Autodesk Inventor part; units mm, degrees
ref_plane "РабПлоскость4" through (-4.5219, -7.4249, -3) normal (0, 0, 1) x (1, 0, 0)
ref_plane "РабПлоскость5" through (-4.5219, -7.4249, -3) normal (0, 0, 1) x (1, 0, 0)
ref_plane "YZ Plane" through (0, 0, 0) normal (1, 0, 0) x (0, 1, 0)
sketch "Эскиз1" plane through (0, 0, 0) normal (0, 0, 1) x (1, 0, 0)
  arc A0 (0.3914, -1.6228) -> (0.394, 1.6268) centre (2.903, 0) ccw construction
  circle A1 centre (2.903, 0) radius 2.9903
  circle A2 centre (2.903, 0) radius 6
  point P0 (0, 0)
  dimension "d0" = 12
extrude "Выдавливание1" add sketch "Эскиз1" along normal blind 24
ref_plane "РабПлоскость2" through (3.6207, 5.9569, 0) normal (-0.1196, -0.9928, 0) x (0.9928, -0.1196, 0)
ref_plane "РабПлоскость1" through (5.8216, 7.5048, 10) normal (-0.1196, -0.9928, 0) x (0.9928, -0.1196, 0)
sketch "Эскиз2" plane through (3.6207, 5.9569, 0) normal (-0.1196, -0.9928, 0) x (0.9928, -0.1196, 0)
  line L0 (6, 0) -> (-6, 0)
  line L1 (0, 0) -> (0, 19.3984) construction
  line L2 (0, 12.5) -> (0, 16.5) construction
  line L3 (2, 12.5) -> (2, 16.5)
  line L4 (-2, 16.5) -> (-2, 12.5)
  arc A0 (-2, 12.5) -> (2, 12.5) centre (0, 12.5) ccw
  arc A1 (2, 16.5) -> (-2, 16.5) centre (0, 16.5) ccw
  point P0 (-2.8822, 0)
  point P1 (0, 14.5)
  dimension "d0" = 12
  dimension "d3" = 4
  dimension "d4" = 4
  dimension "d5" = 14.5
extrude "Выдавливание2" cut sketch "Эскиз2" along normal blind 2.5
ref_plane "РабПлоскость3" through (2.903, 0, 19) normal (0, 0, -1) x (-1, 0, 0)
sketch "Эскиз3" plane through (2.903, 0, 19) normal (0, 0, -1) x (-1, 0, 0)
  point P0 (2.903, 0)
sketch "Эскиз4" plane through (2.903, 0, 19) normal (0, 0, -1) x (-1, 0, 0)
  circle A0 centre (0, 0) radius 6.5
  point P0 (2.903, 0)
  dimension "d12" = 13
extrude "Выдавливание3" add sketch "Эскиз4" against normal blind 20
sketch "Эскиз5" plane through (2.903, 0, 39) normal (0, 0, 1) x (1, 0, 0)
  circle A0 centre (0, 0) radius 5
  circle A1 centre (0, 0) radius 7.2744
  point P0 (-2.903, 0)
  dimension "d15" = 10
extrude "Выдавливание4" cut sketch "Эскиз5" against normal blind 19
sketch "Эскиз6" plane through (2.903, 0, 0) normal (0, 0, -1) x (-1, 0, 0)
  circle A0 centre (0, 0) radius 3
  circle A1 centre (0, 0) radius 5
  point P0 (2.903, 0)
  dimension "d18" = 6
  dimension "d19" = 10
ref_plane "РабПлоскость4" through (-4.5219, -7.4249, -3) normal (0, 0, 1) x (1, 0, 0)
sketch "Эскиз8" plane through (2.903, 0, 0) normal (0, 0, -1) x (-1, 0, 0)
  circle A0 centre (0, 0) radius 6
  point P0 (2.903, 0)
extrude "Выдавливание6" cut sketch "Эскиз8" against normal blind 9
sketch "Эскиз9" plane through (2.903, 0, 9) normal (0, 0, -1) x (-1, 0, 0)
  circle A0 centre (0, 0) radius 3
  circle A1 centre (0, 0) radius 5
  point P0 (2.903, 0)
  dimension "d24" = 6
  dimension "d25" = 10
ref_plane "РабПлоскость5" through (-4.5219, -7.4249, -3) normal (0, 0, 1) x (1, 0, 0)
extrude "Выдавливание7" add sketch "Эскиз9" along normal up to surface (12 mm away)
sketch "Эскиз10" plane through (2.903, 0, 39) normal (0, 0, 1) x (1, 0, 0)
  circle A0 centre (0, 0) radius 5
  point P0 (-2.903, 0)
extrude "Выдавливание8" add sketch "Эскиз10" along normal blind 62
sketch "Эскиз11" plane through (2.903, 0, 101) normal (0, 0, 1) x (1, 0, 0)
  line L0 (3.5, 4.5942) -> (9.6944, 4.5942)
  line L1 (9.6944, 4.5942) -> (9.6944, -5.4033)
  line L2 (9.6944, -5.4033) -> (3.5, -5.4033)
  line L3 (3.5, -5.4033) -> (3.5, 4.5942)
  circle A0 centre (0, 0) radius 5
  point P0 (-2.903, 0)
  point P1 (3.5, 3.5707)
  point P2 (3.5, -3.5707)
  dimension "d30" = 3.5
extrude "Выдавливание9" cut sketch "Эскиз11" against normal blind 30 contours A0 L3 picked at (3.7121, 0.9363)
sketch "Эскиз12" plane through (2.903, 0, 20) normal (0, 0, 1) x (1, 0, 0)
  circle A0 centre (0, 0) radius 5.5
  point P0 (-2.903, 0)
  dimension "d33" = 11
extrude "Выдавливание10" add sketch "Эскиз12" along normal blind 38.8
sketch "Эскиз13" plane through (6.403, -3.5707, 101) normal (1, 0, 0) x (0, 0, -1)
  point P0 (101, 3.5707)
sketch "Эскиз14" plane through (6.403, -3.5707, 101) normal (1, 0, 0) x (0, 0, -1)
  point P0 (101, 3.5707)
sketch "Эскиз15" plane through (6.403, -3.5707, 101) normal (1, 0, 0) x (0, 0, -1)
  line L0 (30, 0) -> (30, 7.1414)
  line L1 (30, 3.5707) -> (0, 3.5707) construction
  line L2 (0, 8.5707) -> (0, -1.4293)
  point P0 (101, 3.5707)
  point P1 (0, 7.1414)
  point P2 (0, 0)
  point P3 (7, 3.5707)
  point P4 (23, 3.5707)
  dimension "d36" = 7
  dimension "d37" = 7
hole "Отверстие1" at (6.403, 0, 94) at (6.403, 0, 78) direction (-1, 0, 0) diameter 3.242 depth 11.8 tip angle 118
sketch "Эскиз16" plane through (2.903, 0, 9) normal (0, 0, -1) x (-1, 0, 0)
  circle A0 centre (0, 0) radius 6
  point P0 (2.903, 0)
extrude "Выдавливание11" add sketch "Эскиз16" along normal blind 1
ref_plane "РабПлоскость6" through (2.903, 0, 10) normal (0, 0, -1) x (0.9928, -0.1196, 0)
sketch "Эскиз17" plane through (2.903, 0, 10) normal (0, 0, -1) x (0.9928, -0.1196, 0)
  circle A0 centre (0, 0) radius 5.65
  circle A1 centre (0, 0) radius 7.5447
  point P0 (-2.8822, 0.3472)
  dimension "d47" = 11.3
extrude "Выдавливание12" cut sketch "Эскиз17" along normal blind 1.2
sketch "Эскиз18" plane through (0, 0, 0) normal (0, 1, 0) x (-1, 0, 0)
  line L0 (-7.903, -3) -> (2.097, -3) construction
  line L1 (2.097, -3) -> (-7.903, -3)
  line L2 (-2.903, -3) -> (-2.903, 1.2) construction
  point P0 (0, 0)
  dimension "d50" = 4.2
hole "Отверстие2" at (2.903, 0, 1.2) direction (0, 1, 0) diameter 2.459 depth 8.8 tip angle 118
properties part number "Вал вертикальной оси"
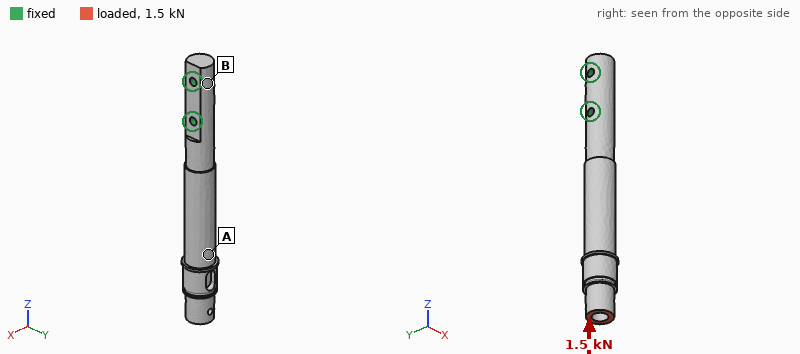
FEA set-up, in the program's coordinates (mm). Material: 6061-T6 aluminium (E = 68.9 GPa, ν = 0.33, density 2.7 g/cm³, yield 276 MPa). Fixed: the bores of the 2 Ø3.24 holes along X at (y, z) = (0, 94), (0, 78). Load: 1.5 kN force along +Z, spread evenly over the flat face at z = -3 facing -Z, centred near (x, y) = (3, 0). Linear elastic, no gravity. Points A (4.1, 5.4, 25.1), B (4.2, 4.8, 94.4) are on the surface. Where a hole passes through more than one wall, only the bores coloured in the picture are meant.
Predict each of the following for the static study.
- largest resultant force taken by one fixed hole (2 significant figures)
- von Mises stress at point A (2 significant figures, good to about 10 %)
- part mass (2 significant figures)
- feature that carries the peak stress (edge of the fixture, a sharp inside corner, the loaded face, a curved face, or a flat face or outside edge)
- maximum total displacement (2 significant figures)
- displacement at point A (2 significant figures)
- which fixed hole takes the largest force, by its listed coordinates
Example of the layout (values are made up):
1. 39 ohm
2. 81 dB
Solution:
1. 1.4 kN
2. 15 MPa
3. 22 g
4. a curved face
5. 32 µm
6. 18 µm
7. (0, 78)
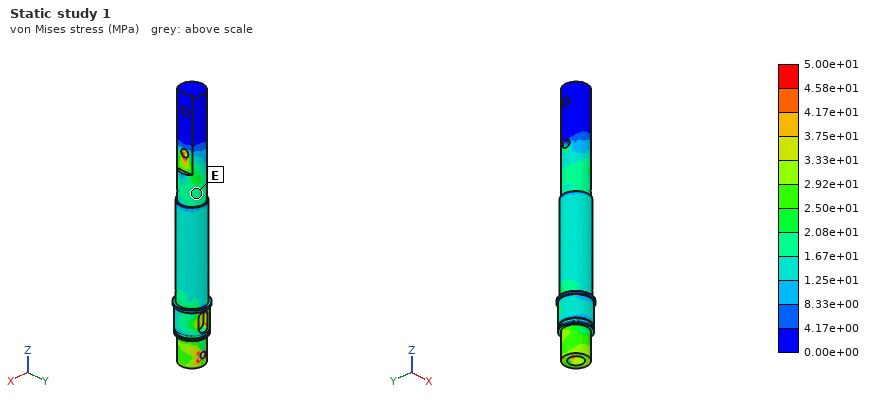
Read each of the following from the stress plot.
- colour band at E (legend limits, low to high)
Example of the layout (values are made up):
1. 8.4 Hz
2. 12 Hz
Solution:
1. 1.67e+01 to 2.08e+01 MPa
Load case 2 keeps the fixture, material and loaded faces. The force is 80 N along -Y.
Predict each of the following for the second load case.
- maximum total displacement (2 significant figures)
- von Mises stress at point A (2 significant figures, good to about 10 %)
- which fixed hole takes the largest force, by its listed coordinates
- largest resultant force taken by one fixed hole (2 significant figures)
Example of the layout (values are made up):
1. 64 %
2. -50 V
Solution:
1. 0.41 mm
2. 16 MPa
3. (0, 78)
4. 240 N
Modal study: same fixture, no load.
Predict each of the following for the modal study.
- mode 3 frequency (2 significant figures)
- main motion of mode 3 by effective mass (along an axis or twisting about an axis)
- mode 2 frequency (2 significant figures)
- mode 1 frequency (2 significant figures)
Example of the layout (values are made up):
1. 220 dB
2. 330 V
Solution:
1. 6900 Hz
2. along Y
3. 1100 Hz
4. 1100 Hz
